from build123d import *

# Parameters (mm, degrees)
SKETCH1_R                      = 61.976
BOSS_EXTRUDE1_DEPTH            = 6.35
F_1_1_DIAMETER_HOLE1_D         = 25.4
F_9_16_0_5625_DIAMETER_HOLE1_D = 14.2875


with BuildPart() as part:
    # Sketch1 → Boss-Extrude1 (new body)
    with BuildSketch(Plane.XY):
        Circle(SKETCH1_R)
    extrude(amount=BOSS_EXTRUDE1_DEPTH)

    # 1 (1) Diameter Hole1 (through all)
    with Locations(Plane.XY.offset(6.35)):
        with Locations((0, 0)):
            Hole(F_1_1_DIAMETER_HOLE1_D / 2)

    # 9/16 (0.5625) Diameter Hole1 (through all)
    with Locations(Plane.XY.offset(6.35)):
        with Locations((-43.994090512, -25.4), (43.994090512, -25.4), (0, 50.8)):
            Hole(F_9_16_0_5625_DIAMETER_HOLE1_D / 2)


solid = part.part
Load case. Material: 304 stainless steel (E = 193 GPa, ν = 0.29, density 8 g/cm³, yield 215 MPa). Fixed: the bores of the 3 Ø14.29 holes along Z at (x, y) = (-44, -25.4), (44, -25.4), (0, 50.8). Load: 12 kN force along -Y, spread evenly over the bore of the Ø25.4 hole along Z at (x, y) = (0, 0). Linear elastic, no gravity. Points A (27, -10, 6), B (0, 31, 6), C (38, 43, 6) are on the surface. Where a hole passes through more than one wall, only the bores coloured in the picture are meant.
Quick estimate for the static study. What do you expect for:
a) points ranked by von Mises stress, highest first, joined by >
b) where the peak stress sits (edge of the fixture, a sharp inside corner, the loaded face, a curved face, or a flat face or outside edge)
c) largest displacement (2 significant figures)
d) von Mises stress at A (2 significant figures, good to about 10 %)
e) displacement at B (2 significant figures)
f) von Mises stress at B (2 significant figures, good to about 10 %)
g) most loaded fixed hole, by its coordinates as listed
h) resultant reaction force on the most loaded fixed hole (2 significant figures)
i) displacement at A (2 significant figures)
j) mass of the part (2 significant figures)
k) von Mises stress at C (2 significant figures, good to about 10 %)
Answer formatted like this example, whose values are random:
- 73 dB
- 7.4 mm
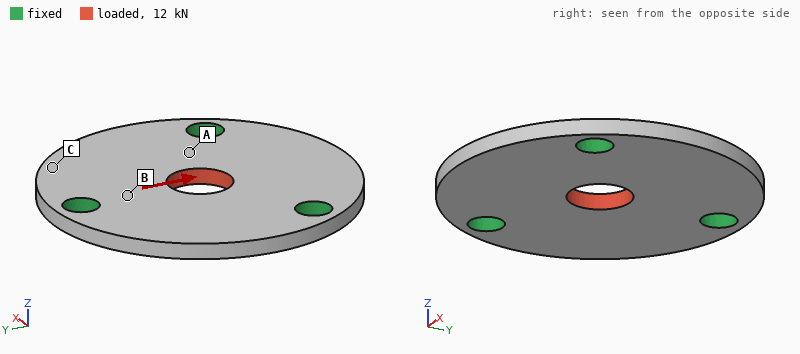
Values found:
- B > A > C
- edge of the fixture
- 6.6 µm
- 13 MPa
- 1.8 µm
- 28 MPa
- (0, 50.8)
- 4.3 kN
- 2.6 µm
- 560 g
- 5.6 MPa
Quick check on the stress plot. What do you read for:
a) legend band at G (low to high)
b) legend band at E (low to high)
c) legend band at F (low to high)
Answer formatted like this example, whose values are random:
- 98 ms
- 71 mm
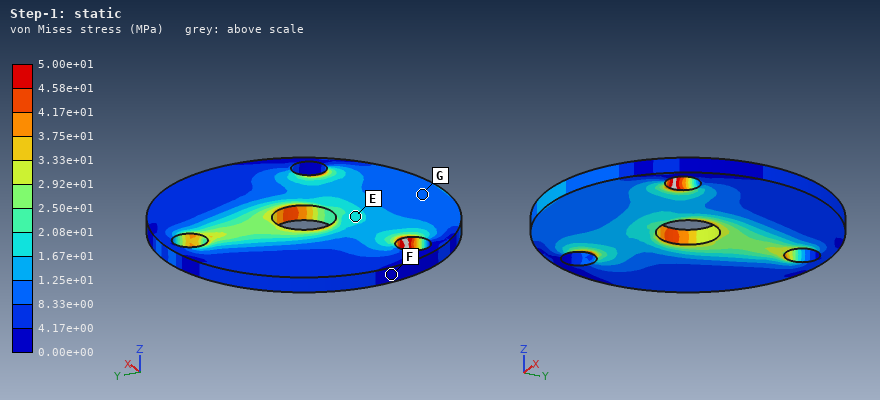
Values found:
- 8.33e+00 to 1.25e+01 MPa
- 1.67e+01 to 2.08e+01 MPa
- 0.00e+00 to 4.17e+00 MPa
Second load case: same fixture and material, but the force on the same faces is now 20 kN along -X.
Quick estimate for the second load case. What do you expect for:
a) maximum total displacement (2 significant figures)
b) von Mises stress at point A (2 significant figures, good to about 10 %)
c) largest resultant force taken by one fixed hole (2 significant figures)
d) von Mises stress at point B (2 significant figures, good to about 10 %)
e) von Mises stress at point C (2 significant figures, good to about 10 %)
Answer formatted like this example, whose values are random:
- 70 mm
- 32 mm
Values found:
- 11 µm
- 39 MPa
- 7.0 kN
- 14 MPa
- 16 MPa
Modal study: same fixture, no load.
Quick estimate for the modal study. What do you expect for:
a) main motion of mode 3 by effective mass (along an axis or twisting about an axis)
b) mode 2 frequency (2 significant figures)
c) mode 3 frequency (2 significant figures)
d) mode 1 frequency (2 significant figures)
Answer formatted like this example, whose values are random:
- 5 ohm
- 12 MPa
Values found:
- along Z
- 3300 Hz
- 3600 Hz
- 3300 Hz
